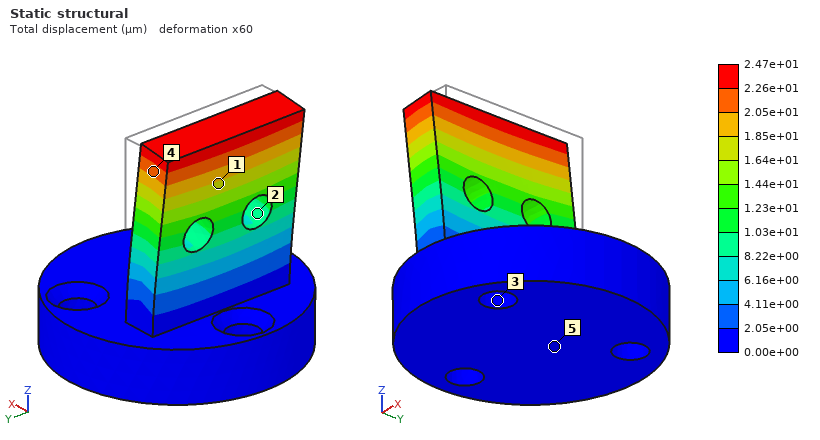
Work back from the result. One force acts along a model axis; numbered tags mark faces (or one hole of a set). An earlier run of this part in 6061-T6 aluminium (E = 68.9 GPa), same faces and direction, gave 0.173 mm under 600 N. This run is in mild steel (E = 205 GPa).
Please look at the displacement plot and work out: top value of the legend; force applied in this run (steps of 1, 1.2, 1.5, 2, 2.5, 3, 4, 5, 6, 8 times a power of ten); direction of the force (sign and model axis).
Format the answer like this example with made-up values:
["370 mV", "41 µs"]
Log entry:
["2.47e+01 µm", "250 N", "-X"]
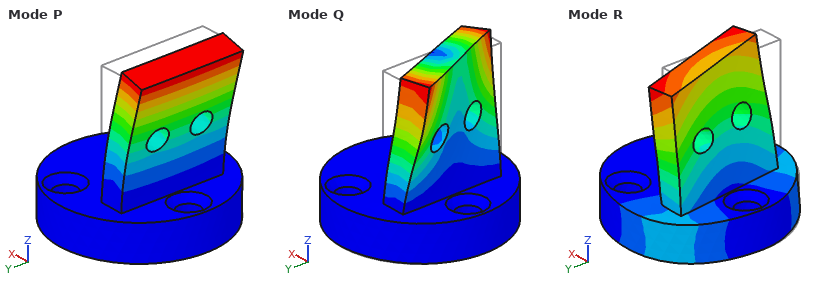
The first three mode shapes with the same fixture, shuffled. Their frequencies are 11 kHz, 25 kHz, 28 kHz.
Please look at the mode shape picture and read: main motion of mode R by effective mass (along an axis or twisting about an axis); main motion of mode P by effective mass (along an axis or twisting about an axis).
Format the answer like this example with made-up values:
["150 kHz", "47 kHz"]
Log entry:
["along Y", "along X"]
